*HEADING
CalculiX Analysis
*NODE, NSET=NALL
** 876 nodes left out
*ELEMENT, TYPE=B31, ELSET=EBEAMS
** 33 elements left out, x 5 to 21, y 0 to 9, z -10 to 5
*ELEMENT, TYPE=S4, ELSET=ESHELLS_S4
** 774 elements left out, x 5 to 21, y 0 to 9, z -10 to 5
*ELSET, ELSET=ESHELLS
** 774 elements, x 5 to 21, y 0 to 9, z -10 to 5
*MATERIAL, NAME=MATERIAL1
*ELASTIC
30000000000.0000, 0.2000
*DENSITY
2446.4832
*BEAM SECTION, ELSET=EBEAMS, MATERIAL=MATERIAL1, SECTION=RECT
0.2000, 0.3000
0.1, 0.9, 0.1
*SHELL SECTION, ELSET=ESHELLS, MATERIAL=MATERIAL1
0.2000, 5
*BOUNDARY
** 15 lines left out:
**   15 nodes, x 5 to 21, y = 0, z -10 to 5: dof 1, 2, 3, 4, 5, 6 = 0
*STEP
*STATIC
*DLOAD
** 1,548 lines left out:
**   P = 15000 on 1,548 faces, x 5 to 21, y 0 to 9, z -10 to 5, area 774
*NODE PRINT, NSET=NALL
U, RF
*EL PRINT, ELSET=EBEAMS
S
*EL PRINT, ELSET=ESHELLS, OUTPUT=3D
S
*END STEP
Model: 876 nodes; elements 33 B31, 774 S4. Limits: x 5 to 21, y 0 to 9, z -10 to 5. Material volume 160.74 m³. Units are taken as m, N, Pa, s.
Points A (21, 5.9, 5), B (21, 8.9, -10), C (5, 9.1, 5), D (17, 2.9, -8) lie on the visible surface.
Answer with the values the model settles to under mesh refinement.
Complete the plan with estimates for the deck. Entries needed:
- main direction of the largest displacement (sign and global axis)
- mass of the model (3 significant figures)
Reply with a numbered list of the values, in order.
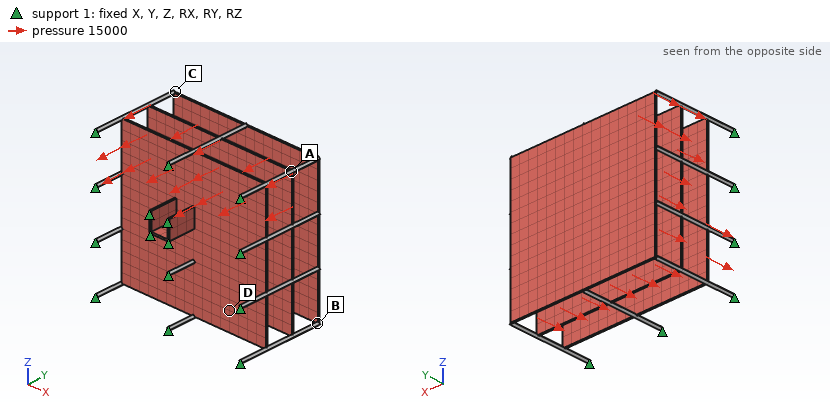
1. -Y
2. 3.93e+05 kg
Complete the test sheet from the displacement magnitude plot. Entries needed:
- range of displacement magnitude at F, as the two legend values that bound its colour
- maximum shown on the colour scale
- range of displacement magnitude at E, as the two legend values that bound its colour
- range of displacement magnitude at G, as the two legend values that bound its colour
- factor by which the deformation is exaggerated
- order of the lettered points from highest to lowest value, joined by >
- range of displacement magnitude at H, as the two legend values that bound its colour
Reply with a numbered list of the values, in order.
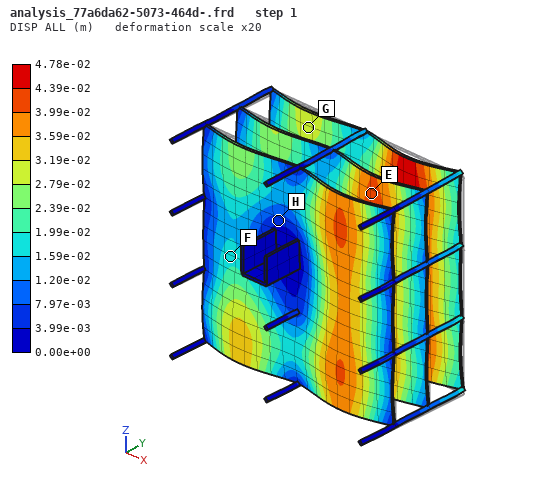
1. 1.59e-02 to 1.99e-02 m
2. 4.78e-02 m
3. 3.99e-02 to 4.39e-02 m
4. 2.79e-02 to 3.19e-02 m
5. 20
6. E > G > F > H
7. 3.99e-03 to 7.97e-03 m
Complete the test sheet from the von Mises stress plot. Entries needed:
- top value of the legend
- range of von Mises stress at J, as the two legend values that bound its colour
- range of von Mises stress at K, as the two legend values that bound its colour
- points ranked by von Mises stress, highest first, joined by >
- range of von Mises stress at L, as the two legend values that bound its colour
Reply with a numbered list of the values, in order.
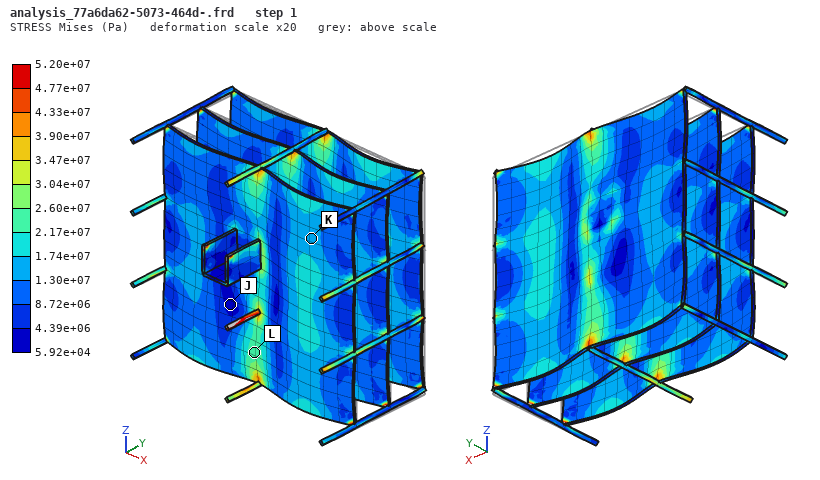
1. 5.20e+07 Pa
2. 5.92e+04 to 4.39e+06 Pa
3. 1.30e+07 to 1.74e+07 Pa
4. L > K > J
5. 2.17e+07 to 2.60e+07 Pa
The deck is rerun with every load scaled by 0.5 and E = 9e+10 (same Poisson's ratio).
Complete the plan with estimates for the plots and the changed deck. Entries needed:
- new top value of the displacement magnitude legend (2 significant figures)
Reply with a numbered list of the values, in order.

1. 0.0080 m
